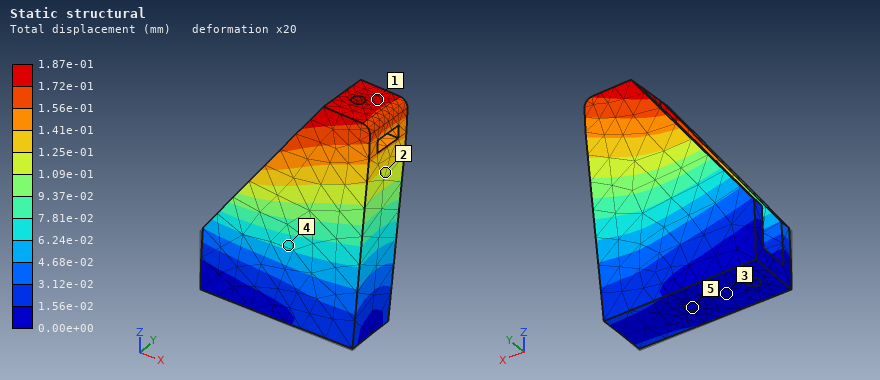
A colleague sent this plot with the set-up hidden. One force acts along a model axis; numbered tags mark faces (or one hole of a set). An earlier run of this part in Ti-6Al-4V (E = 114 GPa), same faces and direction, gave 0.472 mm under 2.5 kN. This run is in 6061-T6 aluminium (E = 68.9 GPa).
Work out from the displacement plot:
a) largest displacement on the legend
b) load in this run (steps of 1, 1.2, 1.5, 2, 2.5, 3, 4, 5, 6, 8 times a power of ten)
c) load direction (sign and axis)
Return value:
1.87e-01 mm
600 N
+Y
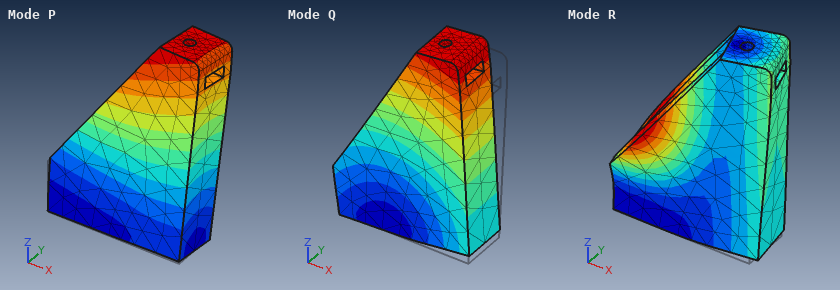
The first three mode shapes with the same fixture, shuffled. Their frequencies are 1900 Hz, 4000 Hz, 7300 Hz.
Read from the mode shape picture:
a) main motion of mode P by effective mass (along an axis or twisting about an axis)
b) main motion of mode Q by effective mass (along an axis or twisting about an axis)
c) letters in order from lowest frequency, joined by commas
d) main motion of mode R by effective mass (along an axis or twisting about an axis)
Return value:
along Y
along X
P, Q, R
twisting about Z
